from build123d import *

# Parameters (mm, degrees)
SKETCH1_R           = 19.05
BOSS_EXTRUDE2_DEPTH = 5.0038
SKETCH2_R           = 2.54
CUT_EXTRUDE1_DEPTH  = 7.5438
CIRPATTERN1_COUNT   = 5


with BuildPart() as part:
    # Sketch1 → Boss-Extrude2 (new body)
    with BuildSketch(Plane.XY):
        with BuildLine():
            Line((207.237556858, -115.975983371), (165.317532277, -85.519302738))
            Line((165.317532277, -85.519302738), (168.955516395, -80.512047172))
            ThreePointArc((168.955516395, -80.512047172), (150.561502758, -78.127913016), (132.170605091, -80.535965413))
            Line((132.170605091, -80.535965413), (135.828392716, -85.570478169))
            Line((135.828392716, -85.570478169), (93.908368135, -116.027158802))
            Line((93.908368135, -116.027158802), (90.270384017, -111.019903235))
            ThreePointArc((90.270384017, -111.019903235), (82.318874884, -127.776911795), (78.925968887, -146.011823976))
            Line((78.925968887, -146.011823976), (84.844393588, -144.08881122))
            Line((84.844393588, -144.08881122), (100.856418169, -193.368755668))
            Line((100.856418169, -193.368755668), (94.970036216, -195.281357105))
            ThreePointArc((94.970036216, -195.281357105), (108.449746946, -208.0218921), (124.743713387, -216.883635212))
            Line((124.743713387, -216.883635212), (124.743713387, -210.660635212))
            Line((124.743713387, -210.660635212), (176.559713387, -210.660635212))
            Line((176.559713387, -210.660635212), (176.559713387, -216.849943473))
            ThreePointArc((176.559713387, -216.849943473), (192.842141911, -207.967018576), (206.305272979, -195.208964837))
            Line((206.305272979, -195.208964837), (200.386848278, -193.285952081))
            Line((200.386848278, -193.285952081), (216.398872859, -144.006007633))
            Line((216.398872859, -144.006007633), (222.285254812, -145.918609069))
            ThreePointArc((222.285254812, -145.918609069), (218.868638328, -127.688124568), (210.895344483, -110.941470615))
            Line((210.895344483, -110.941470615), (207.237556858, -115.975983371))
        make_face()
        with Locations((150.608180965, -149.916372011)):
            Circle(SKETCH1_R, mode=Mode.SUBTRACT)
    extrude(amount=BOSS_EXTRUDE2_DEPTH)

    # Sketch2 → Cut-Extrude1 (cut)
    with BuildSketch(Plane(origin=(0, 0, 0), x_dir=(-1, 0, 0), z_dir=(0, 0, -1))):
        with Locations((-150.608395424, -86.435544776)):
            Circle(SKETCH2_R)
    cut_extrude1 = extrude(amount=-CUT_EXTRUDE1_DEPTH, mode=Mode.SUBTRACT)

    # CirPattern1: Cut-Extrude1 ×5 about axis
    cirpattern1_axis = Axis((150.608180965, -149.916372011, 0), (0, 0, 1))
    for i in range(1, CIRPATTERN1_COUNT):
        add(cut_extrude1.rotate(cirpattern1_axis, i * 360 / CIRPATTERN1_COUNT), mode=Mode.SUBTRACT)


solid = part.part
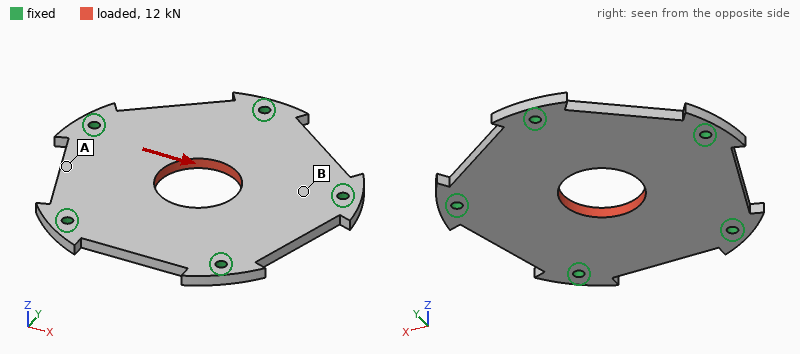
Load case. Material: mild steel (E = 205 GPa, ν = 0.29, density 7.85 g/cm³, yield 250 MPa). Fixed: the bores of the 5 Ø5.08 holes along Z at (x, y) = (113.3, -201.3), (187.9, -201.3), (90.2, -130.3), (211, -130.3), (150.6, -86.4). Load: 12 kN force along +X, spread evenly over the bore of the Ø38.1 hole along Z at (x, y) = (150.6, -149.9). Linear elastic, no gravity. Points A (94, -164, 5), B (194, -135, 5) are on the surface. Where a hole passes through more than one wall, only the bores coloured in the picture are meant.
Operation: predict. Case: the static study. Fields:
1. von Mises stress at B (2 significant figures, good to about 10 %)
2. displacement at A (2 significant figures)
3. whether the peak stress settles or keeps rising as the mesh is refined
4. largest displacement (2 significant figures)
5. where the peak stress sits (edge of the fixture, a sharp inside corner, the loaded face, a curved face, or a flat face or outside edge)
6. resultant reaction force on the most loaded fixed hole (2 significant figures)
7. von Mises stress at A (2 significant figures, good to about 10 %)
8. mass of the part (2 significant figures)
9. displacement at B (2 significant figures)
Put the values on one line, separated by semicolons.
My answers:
29 MPa; 4.4 µm; keeps rising; 6.4 µm; edge of the fixture; 3.4 kN; 11 MPa; 490 g; 2.9 µm
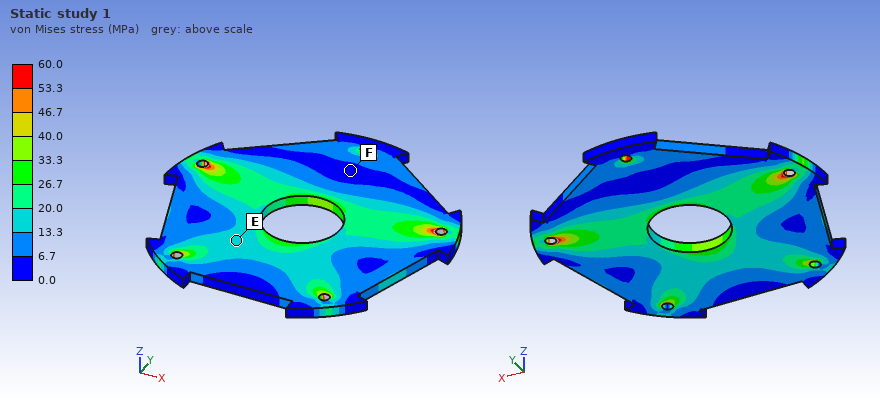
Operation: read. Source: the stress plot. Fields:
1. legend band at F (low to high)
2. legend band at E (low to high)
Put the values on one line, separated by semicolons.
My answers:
0.0 to 6.7 MPa; 13.3 to 20.0 MPa
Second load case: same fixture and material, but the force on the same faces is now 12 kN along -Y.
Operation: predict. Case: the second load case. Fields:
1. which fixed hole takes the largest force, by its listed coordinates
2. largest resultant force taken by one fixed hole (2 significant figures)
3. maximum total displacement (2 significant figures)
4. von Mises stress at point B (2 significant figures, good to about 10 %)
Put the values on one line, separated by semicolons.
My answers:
(150.6, -86.4); 3.5 kN; 6.4 µm; 11 MPa
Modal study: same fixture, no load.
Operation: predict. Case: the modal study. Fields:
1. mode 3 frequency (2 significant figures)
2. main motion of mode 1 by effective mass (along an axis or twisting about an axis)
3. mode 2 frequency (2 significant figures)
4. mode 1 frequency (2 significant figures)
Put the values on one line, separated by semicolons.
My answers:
4200 Hz; along Z; 4200 Hz; 2500 Hz
